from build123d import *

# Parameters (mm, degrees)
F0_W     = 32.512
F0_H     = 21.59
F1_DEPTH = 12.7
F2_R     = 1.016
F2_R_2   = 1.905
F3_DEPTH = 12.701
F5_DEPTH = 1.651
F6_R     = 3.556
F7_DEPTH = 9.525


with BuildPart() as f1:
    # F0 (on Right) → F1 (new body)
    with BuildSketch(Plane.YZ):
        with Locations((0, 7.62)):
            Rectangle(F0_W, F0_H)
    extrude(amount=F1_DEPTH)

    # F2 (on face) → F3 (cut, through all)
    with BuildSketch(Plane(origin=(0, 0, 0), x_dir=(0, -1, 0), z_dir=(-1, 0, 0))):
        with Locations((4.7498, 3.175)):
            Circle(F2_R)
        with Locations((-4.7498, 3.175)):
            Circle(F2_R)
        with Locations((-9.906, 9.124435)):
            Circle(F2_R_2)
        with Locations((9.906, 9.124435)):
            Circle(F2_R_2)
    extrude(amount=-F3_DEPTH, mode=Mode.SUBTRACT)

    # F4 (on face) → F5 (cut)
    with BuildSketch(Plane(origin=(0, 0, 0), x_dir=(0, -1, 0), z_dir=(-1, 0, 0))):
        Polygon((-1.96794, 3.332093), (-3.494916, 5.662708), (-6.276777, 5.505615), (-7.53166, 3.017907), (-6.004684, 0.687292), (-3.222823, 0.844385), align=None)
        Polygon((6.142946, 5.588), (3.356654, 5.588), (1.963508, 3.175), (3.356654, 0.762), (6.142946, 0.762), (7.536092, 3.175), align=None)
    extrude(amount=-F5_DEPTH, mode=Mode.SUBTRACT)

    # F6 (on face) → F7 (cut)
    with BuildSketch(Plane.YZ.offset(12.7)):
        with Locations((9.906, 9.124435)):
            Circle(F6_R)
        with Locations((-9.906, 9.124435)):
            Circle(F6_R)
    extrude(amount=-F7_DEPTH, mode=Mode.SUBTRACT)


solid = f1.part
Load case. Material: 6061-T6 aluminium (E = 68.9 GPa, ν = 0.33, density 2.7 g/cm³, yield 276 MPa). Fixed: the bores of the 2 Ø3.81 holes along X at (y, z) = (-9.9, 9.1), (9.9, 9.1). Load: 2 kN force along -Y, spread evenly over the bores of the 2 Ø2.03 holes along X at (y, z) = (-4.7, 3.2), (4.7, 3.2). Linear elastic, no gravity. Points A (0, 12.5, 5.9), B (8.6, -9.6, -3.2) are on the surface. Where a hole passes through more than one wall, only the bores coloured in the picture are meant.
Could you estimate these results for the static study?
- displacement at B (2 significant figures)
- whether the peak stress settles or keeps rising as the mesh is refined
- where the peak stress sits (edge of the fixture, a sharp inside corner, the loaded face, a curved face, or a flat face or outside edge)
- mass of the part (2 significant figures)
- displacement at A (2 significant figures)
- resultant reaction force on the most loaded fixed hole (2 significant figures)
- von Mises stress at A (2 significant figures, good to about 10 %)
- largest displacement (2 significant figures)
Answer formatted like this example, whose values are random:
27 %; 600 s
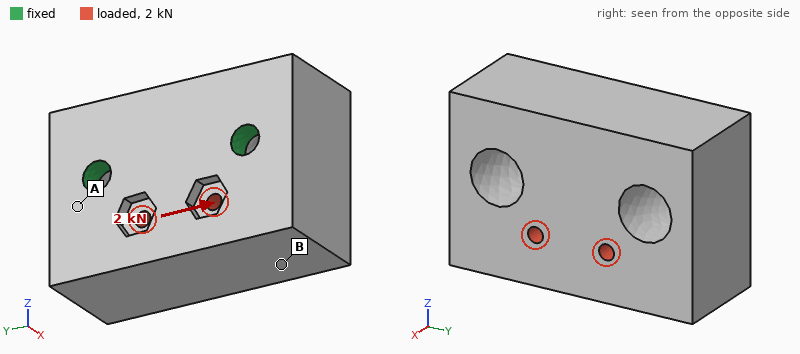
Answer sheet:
6.1 µm; keeps rising; edge of the fixture; 21 g; 2.1 µm; 1.2 kN; 18 MPa; 7.5 µm
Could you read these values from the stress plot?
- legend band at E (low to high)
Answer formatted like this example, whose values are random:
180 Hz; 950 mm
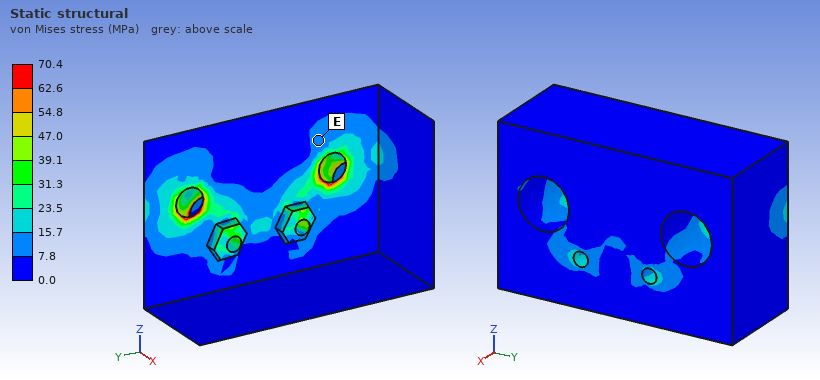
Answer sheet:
7.8 to 15.7 MPa
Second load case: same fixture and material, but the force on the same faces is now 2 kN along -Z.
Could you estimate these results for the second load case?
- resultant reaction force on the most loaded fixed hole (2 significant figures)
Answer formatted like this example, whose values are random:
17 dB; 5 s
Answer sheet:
1.0 kN
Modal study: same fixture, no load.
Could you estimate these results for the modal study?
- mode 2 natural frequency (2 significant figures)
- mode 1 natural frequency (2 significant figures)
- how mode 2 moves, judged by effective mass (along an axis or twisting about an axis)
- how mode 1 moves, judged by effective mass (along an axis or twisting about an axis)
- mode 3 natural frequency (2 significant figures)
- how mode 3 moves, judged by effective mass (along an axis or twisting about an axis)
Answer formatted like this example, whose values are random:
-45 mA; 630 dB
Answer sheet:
23 kHz; 8700 Hz; along Y; along Z; 24 kHz; twisting about X
